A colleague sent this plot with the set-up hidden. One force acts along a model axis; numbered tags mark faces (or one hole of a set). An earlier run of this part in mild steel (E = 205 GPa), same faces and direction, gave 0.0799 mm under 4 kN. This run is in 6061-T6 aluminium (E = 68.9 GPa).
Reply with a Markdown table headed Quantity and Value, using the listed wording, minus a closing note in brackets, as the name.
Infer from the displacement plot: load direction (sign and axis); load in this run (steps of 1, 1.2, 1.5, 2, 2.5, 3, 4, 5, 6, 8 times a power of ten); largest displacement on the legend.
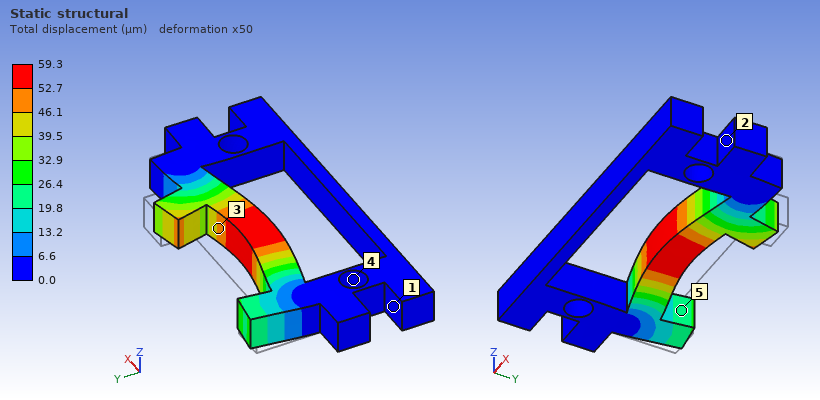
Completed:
| Quantity | Value |
|---|---|
| load direction | -Y |
| load in this run | 1 kN |
| largest displacement on the legend | 59.3 µm |
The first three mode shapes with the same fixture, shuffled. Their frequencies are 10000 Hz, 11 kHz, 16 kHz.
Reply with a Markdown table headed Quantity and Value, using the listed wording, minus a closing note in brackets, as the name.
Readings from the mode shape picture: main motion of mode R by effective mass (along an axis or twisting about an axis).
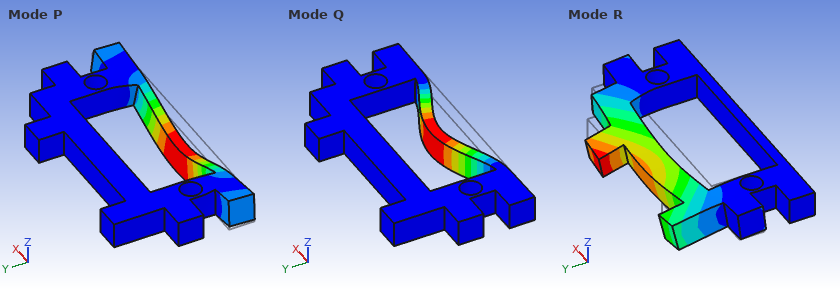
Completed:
| Quantity | Value |
|---|---|
| main motion of mode R by effective mass | along Z |
